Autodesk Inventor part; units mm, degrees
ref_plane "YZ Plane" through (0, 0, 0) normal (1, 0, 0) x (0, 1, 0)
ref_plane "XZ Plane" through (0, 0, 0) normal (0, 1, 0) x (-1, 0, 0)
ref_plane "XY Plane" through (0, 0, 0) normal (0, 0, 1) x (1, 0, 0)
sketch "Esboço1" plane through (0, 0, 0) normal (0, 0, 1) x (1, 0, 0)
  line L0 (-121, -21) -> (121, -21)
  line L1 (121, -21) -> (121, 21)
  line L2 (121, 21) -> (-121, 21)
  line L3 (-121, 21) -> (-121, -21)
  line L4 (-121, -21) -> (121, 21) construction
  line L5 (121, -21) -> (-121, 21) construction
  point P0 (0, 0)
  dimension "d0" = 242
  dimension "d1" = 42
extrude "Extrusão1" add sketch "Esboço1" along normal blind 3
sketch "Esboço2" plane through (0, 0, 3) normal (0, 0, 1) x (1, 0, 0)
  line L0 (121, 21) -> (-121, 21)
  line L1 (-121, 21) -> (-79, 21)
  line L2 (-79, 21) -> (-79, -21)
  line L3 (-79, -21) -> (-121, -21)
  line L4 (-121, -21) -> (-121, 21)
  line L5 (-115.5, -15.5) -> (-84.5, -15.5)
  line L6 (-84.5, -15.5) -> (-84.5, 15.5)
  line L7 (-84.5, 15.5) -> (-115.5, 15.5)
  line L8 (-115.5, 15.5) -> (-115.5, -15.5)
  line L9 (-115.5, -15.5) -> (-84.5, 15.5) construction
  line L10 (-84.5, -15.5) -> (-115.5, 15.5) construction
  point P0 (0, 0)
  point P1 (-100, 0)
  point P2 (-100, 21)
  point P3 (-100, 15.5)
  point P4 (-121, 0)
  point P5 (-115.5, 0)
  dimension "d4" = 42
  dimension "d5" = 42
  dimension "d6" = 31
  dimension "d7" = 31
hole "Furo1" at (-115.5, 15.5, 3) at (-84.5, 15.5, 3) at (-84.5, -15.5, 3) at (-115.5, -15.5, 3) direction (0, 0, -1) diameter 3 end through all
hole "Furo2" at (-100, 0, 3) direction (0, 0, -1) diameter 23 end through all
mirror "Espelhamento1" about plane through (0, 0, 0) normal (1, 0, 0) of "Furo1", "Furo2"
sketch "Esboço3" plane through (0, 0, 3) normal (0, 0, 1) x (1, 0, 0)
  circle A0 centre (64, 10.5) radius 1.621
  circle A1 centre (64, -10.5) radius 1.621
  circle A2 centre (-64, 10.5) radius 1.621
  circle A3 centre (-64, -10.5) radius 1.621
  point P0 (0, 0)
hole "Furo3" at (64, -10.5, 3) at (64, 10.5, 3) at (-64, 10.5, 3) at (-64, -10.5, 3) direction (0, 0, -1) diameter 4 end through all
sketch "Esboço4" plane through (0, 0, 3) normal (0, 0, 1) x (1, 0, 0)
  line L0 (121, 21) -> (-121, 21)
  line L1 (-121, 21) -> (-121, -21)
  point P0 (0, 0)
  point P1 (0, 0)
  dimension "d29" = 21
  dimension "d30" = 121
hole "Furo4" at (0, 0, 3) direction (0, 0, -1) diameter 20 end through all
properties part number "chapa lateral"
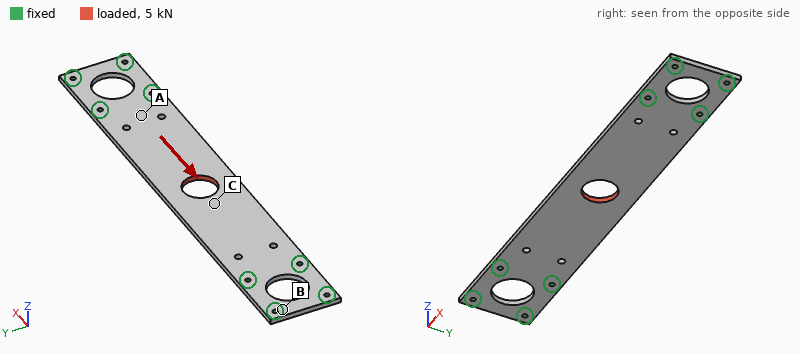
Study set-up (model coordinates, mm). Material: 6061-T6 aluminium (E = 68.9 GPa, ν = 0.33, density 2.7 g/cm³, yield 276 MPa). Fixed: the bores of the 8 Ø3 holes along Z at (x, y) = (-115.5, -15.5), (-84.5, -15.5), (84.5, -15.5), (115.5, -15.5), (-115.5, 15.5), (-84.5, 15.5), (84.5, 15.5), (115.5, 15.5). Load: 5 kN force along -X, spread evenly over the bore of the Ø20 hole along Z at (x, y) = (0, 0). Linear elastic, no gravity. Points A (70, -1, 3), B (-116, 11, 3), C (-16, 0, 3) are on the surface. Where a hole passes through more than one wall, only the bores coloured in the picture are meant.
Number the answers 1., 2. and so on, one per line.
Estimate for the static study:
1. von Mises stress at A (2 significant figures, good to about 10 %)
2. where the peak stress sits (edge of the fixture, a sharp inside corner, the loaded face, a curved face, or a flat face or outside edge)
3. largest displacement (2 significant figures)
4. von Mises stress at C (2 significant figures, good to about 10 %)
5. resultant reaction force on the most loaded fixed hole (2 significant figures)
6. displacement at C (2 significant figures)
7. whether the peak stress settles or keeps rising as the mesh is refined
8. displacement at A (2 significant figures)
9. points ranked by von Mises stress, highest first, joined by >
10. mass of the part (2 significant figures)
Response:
1. 15 MPa
2. edge of the fixture
3. 28 µm
4. 27 MPa
5. 1.2 kN
6. 24 µm
7. keeps rising
8. 7.6 µm
9. C > A > B
10. 72 g
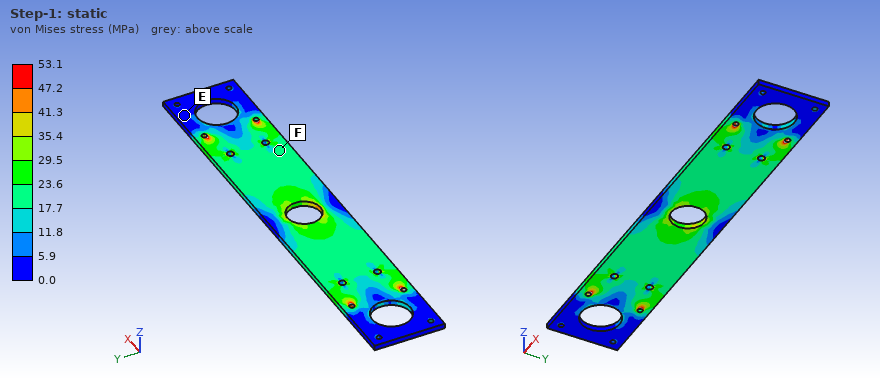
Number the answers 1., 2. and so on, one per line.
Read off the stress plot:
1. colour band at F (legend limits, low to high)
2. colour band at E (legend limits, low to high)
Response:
1. 17.7 to 23.6 MPa
2. 0.0 to 5.9 MPa
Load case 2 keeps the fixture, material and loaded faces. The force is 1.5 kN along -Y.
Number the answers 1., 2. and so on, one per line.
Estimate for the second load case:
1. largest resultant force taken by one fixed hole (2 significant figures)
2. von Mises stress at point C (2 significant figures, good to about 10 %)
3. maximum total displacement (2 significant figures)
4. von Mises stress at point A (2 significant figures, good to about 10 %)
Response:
1. 980 N
2. 14 MPa
3. 55 µm
4. 14 MPa
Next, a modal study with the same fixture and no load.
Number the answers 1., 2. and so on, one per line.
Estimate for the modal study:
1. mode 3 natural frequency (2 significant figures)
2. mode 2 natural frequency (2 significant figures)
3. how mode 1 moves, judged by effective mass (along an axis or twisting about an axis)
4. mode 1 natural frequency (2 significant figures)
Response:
1. 1500 Hz
2. 1500 Hz
3. along Z
4. 530 Hz
